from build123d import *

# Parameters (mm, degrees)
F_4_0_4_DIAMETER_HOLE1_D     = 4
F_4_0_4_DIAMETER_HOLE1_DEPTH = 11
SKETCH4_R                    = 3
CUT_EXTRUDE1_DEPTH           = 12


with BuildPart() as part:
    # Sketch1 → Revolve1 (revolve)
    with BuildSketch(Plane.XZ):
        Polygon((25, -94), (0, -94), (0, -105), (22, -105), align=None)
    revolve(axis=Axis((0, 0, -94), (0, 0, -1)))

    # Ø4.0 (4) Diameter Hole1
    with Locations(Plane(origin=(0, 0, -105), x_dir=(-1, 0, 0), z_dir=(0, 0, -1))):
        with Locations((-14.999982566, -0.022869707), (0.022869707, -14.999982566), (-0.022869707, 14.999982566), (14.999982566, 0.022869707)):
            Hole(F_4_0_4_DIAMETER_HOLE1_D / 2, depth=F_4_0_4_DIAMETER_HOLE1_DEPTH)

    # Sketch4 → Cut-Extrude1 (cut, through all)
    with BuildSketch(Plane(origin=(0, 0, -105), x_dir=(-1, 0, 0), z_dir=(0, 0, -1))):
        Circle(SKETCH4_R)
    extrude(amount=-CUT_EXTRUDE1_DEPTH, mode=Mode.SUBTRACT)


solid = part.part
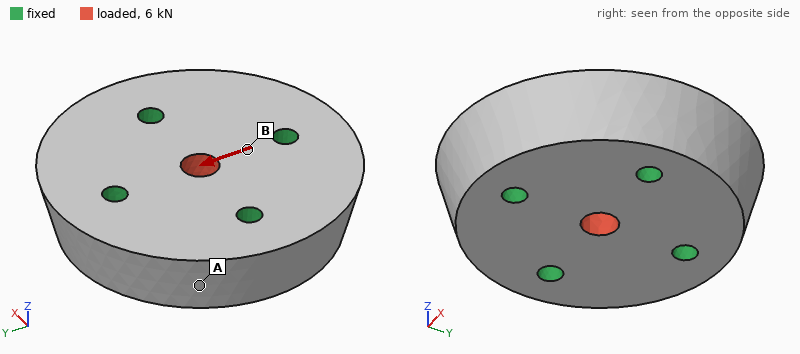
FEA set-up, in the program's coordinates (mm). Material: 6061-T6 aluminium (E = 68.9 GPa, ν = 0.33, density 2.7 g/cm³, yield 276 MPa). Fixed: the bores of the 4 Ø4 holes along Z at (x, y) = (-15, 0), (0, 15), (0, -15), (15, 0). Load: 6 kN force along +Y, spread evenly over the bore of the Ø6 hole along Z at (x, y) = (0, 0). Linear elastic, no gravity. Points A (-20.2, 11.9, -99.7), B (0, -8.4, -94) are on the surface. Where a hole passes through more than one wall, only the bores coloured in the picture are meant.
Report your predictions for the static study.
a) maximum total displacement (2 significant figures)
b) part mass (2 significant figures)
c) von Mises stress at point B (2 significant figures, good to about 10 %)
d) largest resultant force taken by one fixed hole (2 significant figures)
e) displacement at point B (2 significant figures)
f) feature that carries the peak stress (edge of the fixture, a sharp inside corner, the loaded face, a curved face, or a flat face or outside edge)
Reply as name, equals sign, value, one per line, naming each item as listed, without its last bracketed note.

maximum total displacement = 4.0 µm
part mass = 49 g
von Mises stress at point B = 25 MPa
largest resultant force taken by one fixed hole = 2.0 kN
displacement at point B = 1.8 µm
feature that carries the peak stress = the loaded face
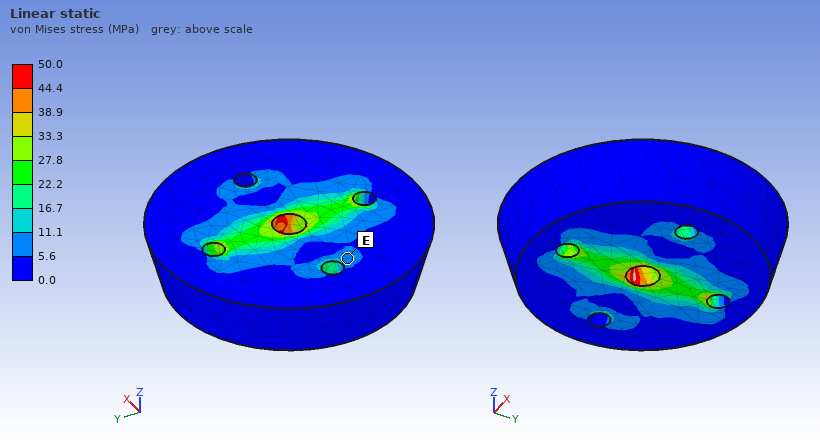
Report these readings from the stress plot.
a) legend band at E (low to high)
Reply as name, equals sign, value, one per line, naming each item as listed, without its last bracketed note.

legend band at E = 5.6 to 11.1 MPa
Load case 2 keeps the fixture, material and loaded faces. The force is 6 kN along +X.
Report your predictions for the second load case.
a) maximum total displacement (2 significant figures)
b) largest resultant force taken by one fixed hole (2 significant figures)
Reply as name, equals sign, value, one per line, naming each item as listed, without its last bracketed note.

maximum total displacement = 4.0 µm
largest resultant force taken by one fixed hole = 2.0 kN
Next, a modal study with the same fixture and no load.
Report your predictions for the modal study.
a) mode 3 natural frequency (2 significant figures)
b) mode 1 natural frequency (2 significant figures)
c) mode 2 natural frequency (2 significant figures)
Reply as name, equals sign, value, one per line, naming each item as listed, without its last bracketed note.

mode 3 natural frequency = 39 kHz
mode 1 natural frequency = 37 kHz
mode 2 natural frequency = 39 kHz
